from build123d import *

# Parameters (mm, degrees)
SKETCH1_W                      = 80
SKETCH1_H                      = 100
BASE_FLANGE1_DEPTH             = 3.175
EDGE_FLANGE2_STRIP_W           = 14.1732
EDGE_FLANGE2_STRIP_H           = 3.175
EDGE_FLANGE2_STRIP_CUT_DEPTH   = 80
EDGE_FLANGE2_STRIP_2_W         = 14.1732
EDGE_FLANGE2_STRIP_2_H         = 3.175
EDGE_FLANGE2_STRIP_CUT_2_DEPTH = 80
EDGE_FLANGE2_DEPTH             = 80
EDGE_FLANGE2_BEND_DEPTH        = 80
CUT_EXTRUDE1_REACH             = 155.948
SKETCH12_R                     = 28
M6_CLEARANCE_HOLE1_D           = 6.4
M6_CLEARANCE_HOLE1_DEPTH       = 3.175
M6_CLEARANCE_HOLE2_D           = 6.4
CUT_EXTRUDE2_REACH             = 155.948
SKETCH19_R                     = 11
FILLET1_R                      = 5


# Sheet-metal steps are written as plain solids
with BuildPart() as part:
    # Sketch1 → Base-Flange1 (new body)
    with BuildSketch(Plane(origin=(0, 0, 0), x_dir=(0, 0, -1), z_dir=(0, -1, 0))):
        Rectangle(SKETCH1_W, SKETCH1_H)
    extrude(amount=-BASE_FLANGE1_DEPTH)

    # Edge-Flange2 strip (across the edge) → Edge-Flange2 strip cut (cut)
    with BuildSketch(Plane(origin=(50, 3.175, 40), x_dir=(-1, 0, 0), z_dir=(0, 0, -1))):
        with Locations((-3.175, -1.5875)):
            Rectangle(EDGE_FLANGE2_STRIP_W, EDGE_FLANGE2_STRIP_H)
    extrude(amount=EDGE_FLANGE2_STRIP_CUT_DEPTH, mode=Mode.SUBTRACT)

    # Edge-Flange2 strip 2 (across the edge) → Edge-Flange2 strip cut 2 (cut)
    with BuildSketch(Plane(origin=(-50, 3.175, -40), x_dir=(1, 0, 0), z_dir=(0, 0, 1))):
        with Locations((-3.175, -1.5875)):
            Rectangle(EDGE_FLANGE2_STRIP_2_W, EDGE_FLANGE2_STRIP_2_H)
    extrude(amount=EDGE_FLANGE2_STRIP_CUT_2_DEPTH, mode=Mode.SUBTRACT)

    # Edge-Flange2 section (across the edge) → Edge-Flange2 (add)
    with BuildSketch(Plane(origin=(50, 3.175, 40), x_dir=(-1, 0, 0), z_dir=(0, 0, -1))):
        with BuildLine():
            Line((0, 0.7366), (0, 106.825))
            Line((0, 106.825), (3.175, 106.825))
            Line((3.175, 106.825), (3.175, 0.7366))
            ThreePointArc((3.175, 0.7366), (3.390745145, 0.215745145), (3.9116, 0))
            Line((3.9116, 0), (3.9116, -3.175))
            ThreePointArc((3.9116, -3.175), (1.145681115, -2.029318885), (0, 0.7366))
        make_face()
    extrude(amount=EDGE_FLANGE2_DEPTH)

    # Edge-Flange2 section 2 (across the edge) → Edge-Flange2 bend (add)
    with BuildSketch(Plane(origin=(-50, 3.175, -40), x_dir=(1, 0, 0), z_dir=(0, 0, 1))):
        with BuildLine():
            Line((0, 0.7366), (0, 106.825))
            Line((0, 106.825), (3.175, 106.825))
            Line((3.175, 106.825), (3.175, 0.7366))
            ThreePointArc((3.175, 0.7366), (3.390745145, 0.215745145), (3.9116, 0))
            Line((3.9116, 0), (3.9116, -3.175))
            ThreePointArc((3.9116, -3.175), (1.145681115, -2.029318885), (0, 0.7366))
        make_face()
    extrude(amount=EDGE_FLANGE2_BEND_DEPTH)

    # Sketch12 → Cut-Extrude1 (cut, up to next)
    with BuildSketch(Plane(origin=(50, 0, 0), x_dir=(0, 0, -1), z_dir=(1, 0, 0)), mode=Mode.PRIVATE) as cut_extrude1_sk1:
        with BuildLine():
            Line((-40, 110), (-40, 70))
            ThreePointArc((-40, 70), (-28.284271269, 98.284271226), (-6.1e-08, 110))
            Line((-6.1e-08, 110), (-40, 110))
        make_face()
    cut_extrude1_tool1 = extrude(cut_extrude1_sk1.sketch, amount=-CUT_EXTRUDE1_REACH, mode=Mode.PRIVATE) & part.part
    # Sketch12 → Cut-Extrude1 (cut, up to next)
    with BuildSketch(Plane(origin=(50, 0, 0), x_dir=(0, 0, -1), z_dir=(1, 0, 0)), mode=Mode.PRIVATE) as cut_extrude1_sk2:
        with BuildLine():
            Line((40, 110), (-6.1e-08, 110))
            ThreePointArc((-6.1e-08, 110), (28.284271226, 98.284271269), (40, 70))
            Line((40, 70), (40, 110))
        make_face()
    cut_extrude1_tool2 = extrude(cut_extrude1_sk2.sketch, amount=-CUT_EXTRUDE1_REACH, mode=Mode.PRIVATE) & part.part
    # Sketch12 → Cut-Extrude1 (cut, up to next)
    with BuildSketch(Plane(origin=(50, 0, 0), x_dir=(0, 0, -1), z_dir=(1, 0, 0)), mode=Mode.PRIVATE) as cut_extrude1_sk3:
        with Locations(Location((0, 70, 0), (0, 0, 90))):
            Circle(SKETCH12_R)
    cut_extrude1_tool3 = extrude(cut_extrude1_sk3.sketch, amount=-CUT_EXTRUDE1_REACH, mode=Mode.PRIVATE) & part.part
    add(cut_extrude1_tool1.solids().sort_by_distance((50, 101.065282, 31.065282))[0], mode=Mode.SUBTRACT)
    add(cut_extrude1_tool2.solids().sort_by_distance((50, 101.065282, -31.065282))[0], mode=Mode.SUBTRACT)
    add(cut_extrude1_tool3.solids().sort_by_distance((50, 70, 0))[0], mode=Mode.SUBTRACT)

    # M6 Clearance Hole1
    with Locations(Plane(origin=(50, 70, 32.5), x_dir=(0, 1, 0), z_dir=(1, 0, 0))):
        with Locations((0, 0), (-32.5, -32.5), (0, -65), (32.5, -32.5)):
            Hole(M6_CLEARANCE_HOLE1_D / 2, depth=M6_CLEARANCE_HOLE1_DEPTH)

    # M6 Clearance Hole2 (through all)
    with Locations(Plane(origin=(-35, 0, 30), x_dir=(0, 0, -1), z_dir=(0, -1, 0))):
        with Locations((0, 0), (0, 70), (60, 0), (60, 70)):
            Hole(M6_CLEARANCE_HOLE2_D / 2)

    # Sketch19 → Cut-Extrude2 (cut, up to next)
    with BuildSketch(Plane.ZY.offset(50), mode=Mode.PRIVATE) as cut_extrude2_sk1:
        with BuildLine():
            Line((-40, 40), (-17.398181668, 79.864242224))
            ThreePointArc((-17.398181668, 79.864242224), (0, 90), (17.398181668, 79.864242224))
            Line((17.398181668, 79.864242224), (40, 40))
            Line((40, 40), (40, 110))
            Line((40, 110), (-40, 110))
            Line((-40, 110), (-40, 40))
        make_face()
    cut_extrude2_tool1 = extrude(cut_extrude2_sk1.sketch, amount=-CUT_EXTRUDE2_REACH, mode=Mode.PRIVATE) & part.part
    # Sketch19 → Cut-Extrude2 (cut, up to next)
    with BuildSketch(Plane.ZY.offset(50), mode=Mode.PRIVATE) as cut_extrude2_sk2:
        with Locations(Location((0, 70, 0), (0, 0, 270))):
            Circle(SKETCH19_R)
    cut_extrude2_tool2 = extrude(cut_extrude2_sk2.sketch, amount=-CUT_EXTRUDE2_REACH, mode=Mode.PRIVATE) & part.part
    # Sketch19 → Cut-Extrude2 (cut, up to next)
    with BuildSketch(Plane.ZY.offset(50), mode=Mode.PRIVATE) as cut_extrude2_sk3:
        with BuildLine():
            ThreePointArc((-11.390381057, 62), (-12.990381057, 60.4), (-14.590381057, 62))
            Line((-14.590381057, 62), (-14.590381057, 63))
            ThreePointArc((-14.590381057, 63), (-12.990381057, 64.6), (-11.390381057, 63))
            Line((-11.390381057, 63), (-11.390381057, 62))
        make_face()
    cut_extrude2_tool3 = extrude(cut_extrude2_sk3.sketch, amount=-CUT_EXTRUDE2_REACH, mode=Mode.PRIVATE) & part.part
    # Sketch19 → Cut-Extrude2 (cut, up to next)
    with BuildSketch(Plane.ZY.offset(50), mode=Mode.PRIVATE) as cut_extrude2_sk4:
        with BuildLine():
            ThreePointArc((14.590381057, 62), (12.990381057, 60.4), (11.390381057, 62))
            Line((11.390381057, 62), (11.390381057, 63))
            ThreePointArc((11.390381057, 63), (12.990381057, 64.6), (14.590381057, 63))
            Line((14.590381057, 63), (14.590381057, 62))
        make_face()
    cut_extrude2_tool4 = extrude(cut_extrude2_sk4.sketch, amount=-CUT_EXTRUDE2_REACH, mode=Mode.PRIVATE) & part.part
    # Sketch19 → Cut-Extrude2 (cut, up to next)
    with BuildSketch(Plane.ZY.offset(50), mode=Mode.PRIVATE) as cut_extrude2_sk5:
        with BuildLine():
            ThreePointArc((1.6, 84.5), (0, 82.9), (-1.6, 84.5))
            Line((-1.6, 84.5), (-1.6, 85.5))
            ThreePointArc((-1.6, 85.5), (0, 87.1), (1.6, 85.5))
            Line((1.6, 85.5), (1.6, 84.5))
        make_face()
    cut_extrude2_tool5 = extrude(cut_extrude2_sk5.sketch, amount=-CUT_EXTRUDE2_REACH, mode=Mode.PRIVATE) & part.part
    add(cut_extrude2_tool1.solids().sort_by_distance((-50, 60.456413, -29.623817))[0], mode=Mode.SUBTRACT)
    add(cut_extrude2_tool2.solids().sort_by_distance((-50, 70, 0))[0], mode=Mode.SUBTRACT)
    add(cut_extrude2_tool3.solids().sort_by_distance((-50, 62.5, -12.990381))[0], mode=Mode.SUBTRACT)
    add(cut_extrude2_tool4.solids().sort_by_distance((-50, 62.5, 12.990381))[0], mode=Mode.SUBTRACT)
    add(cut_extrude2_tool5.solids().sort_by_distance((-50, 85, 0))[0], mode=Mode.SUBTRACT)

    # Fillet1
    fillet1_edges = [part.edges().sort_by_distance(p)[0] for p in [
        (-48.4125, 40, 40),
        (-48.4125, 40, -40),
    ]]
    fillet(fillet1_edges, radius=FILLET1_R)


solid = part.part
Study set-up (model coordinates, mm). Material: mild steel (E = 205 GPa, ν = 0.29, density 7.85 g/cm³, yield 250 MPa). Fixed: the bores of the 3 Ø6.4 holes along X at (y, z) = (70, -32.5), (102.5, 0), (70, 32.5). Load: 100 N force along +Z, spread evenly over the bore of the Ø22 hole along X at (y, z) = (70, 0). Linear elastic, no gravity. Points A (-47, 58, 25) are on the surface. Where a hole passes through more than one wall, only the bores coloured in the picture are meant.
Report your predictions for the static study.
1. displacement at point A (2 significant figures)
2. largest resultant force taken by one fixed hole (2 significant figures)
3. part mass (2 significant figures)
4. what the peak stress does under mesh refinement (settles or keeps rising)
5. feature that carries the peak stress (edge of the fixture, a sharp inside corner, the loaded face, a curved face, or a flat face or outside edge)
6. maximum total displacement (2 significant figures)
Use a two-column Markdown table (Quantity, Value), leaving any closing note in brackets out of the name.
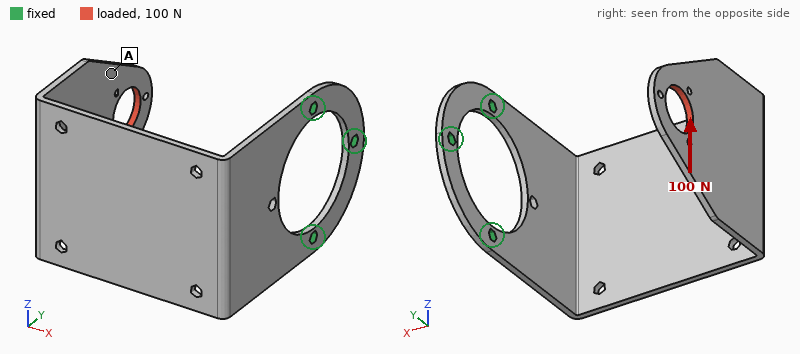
| Quantity | Value |
|---|---|
| displacement at point A | 1.4 mm |
| largest resultant force taken by one fixed hole | 130 N |
| part mass | 450 g |
| what the peak stress does under mesh refinement | keeps rising |
| feature that carries the peak stress | edge of the fixture |
| maximum total displacement | 1.7 mm |
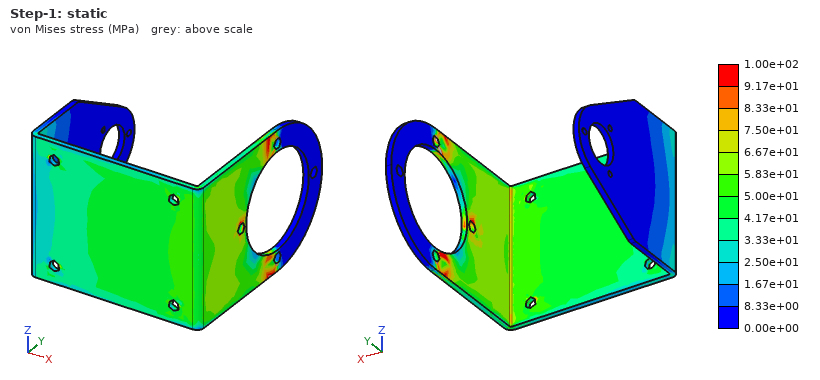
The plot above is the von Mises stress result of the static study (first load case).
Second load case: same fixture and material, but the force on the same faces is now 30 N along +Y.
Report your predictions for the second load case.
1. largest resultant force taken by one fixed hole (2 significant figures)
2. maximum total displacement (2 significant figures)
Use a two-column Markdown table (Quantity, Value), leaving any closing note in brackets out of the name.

| Quantity | Value |
|---|---|
| largest resultant force taken by one fixed hole | 16 N |
| maximum total displacement | 1.1 mm |
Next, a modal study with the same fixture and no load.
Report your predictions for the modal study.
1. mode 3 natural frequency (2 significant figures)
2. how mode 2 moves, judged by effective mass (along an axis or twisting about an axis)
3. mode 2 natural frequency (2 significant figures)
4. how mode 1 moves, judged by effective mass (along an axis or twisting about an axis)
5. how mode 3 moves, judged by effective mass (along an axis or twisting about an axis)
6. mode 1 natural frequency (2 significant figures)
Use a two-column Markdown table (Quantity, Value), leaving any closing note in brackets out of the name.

| Quantity | Value |
|---|---|
| mode 3 natural frequency | 170 Hz |
| how mode 2 moves, judged by effective mass | along Z |
| mode 2 natural frequency | 120 Hz |
| how mode 1 moves, judged by effective mass | along Y |
| how mode 3 moves, judged by effective mass | along X |
| mode 1 natural frequency | 62 Hz |
